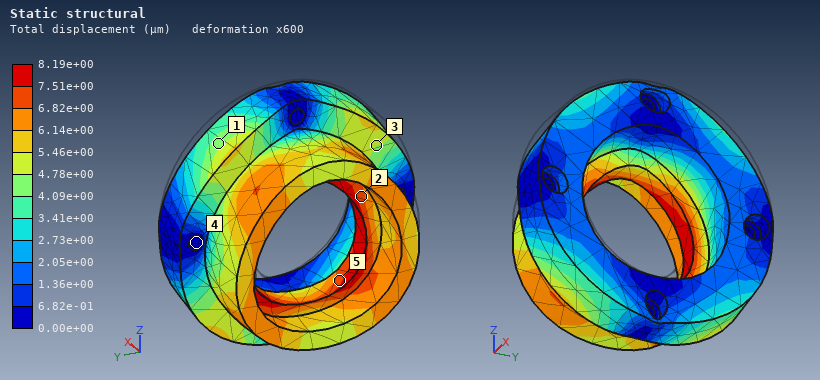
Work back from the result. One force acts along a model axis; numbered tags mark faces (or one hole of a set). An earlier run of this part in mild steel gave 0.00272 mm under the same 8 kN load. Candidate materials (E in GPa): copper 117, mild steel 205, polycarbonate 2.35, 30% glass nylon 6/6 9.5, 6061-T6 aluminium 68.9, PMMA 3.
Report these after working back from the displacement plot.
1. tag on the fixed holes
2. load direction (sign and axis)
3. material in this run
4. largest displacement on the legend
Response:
4
-Z
6061-T6 aluminium
8.19e+00 µm
